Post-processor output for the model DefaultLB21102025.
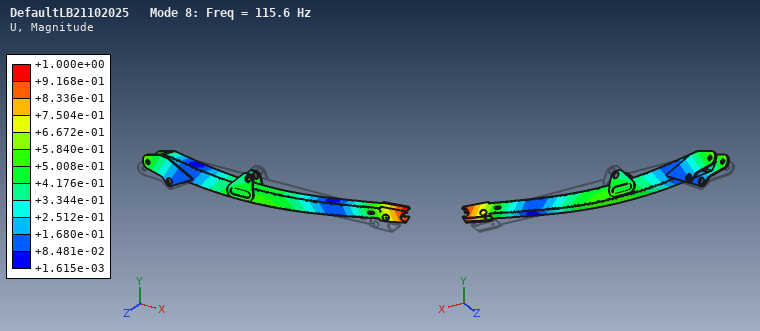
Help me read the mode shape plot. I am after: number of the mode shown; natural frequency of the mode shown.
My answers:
8
115.6 Hz
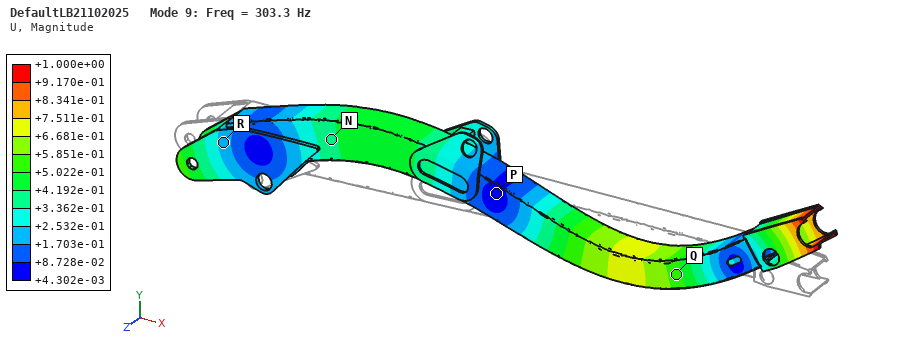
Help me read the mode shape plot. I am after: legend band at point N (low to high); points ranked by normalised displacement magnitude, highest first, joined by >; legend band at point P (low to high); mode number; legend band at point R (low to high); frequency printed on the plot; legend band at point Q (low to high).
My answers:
+3.362e-01 to +4.192e-01
Q > N > R > P
+4.302e-03 to +8.728e-02
9
+1.703e-01 to +2.532e-01
303.3 Hz
+5.022e-01 to +5.851e-01
